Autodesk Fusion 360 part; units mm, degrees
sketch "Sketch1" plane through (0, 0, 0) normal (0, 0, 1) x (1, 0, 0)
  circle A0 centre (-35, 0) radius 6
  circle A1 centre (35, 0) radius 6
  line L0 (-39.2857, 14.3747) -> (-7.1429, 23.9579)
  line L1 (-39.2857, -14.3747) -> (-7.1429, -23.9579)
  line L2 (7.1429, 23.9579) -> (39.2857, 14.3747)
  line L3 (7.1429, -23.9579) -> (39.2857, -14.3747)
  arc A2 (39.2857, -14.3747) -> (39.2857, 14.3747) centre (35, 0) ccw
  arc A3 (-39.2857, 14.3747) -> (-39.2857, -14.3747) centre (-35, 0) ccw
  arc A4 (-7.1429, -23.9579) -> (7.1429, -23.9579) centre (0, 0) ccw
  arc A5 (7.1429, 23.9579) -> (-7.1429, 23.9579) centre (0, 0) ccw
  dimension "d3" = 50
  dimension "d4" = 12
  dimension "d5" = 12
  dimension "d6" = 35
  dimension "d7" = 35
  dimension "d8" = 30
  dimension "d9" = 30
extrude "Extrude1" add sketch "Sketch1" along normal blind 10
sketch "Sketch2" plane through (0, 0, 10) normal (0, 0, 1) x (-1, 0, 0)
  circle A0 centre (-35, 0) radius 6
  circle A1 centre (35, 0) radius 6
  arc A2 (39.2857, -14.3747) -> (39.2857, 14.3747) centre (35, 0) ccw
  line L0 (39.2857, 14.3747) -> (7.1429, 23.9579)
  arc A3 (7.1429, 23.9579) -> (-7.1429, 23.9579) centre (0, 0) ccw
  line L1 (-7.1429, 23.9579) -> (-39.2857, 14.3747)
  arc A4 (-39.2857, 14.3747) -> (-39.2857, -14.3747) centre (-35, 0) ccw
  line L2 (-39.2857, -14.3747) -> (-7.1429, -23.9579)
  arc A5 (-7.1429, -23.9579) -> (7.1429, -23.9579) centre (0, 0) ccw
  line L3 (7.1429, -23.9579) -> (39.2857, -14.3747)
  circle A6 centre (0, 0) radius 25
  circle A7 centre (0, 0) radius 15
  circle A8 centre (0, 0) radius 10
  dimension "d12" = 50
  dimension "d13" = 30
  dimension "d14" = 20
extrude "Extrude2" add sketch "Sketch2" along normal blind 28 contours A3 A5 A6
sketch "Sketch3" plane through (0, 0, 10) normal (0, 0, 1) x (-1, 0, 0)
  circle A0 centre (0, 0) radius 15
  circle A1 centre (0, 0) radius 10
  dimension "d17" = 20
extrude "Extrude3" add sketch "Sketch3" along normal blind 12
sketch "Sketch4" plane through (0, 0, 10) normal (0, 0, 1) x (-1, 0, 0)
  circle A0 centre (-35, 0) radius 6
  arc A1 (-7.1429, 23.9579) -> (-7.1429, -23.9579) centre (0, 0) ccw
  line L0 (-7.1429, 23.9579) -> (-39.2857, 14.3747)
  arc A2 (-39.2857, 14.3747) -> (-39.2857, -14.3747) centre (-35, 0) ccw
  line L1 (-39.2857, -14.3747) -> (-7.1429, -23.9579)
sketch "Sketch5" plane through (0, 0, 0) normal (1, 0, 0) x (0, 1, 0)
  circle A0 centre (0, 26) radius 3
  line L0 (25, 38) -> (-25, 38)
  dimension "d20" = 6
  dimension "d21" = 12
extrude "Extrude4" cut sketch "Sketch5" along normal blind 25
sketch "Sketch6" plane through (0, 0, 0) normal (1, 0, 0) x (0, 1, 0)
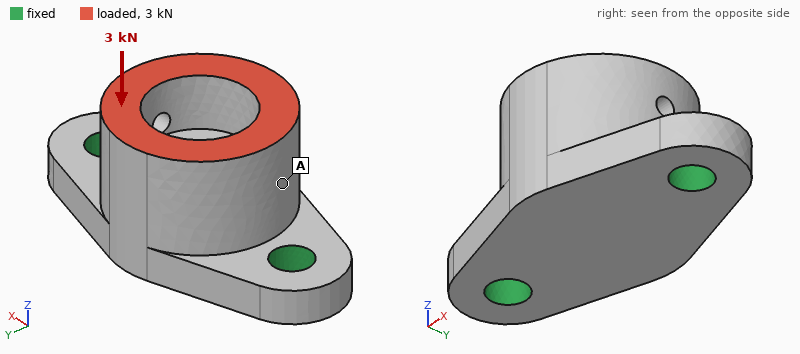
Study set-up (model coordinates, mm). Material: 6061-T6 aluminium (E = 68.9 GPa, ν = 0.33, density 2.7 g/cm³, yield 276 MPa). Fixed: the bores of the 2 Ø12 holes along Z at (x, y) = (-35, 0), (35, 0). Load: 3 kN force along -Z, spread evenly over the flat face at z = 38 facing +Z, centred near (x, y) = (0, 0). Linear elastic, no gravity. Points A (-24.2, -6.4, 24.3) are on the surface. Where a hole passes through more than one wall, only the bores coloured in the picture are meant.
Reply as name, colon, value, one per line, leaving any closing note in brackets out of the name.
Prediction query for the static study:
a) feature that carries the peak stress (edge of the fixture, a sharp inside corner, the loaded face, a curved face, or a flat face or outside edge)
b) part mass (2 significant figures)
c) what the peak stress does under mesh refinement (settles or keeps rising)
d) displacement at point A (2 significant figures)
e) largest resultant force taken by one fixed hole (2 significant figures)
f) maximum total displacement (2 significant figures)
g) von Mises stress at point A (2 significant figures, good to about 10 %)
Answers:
feature that carries the peak stress: edge of the fixture
part mass: 200 g
what the peak stress does under mesh refinement: keeps rising
displacement at point A: 4.7 µm
largest resultant force taken by one fixed hole: 1.6 kN
maximum total displacement: 7.3 µm
von Mises stress at point A: 3.8 MPa
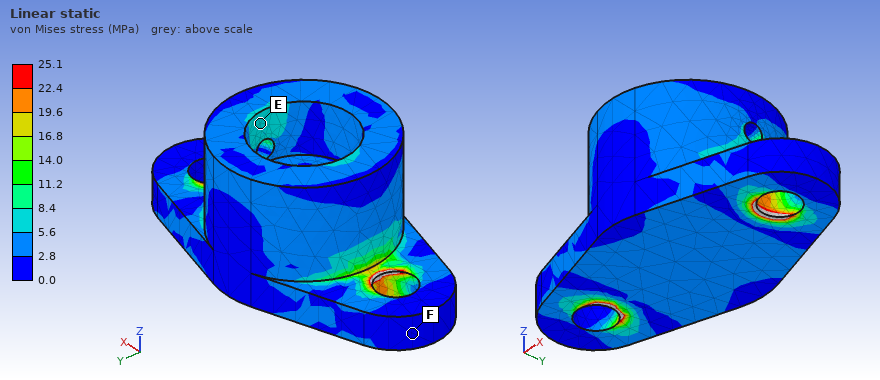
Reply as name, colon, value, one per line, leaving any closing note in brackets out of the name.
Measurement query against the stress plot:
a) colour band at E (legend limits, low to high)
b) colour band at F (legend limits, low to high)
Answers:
colour band at E: 5.6 to 8.4 MPa
colour band at F: 0.0 to 2.8 MPa
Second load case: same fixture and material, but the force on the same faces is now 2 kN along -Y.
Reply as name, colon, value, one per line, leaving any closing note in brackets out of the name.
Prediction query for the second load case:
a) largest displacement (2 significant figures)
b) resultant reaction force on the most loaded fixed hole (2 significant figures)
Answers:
largest displacement: 56 µm
resultant reaction force on the most loaded fixed hole: 1.0 kN
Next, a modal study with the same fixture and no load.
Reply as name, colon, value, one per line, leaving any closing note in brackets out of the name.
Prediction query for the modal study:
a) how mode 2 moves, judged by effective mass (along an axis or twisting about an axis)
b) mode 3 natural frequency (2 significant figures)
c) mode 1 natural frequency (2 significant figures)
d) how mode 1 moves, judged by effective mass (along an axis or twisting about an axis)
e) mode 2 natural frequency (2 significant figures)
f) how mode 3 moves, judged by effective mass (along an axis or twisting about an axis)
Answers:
how mode 2 moves, judged by effective mass: along Z
mode 3 natural frequency: 12 kHz
mode 1 natural frequency: 4200 Hz
how mode 1 moves, judged by effective mass: along Y
mode 2 natural frequency: 9200 Hz
how mode 3 moves, judged by effective mass: along X
